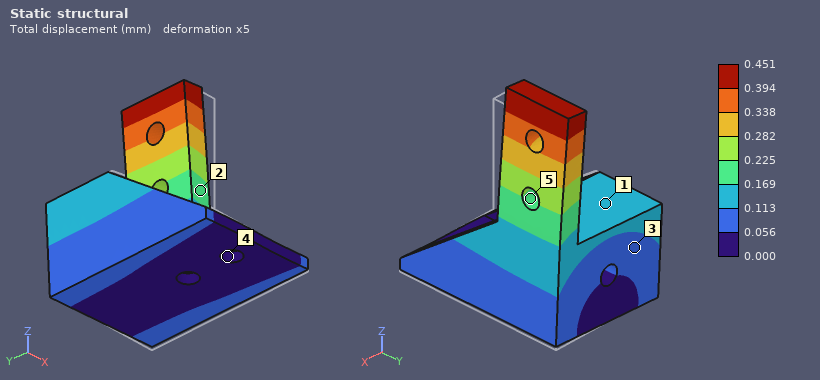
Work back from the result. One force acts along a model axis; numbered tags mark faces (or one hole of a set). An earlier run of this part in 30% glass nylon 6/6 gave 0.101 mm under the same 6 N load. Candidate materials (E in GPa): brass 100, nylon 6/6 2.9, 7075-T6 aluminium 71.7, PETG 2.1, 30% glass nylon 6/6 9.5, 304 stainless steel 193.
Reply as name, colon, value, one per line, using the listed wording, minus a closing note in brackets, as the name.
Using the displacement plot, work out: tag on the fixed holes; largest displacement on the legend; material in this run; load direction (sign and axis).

tag on the fixed holes: 4
largest displacement on the legend: 0.451 mm
material in this run: PETG
load direction: -X
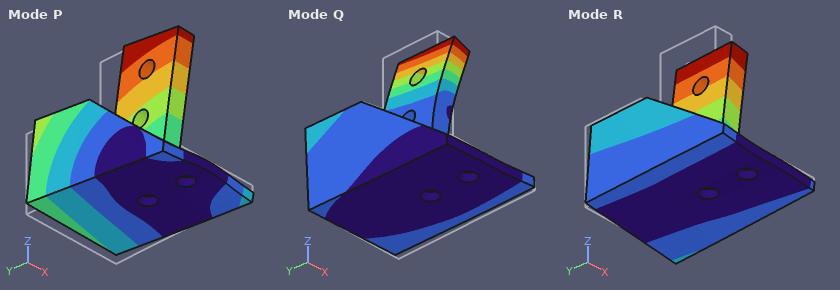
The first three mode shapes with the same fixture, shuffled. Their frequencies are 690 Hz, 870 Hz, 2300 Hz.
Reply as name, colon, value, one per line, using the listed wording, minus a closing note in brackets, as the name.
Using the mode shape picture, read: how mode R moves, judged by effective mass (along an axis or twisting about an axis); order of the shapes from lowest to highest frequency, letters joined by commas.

how mode R moves, judged by effective mass: along X
order of the shapes from lowest to highest frequency, letters joined by commas: R, P, Q
